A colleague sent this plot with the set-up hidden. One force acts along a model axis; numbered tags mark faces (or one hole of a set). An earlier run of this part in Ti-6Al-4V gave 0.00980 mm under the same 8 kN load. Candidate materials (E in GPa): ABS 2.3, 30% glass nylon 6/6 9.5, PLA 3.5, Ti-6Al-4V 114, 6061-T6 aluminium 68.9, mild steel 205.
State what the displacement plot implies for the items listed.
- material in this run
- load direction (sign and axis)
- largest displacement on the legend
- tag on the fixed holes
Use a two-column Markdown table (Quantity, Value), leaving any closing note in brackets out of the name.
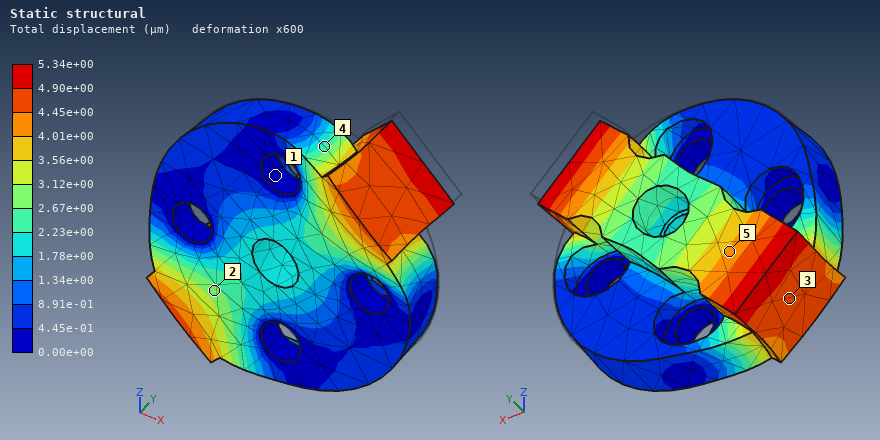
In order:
| Quantity | Value |
|---|---|
| material in this run | mild steel |
| load direction | -Y |
| largest displacement on the legend | 5.34e+00 µm |
| tag on the fixed holes | 1 |
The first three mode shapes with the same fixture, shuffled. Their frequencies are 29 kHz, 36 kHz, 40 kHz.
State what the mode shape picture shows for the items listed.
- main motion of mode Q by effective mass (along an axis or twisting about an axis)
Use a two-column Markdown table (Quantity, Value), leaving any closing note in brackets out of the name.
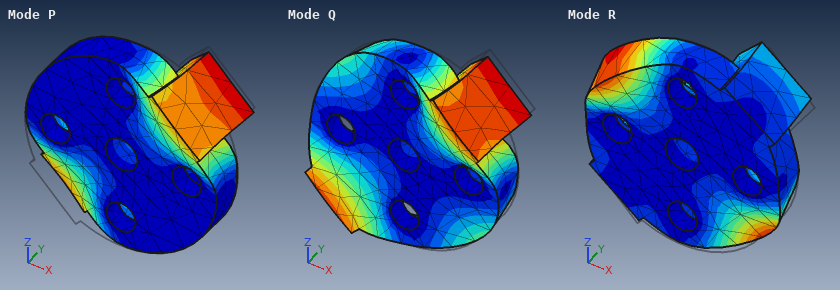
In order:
| Quantity | Value |
|---|---|
| main motion of mode Q by effective mass | along Y |
